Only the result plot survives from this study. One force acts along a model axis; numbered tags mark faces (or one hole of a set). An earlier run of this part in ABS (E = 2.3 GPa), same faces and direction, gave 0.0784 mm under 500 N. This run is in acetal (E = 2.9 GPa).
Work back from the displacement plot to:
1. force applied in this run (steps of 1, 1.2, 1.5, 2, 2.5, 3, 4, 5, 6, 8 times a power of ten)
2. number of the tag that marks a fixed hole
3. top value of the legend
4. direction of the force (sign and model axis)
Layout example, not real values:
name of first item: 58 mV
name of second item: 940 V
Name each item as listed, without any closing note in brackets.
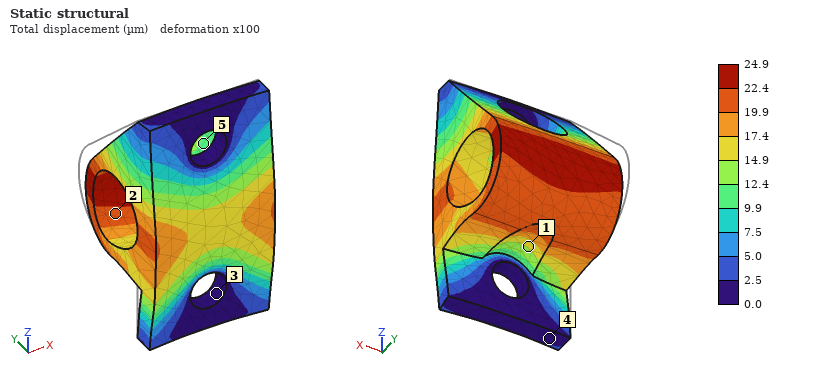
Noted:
force applied in this run: 200 N
number of the tag that marks a fixed hole: 3
top value of the legend: 24.9 µm
direction of the force: -Y
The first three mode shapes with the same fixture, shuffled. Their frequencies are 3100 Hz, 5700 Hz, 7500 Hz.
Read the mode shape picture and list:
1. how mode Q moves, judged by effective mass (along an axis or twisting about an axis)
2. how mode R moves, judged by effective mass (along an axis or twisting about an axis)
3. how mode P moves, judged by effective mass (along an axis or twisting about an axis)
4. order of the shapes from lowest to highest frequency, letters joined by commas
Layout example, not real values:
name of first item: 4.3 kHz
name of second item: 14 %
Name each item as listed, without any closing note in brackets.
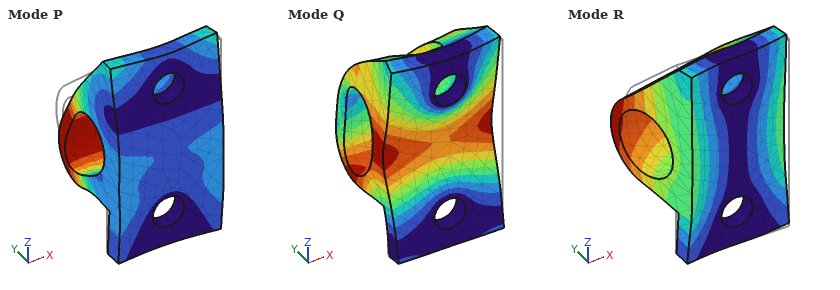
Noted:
how mode Q moves, judged by effective mass: along Y
how mode R moves, judged by effective mass: along X
how mode P moves, judged by effective mass: along Z
order of the shapes from lowest to highest frequency, letters joined by commas: R, P, Q
